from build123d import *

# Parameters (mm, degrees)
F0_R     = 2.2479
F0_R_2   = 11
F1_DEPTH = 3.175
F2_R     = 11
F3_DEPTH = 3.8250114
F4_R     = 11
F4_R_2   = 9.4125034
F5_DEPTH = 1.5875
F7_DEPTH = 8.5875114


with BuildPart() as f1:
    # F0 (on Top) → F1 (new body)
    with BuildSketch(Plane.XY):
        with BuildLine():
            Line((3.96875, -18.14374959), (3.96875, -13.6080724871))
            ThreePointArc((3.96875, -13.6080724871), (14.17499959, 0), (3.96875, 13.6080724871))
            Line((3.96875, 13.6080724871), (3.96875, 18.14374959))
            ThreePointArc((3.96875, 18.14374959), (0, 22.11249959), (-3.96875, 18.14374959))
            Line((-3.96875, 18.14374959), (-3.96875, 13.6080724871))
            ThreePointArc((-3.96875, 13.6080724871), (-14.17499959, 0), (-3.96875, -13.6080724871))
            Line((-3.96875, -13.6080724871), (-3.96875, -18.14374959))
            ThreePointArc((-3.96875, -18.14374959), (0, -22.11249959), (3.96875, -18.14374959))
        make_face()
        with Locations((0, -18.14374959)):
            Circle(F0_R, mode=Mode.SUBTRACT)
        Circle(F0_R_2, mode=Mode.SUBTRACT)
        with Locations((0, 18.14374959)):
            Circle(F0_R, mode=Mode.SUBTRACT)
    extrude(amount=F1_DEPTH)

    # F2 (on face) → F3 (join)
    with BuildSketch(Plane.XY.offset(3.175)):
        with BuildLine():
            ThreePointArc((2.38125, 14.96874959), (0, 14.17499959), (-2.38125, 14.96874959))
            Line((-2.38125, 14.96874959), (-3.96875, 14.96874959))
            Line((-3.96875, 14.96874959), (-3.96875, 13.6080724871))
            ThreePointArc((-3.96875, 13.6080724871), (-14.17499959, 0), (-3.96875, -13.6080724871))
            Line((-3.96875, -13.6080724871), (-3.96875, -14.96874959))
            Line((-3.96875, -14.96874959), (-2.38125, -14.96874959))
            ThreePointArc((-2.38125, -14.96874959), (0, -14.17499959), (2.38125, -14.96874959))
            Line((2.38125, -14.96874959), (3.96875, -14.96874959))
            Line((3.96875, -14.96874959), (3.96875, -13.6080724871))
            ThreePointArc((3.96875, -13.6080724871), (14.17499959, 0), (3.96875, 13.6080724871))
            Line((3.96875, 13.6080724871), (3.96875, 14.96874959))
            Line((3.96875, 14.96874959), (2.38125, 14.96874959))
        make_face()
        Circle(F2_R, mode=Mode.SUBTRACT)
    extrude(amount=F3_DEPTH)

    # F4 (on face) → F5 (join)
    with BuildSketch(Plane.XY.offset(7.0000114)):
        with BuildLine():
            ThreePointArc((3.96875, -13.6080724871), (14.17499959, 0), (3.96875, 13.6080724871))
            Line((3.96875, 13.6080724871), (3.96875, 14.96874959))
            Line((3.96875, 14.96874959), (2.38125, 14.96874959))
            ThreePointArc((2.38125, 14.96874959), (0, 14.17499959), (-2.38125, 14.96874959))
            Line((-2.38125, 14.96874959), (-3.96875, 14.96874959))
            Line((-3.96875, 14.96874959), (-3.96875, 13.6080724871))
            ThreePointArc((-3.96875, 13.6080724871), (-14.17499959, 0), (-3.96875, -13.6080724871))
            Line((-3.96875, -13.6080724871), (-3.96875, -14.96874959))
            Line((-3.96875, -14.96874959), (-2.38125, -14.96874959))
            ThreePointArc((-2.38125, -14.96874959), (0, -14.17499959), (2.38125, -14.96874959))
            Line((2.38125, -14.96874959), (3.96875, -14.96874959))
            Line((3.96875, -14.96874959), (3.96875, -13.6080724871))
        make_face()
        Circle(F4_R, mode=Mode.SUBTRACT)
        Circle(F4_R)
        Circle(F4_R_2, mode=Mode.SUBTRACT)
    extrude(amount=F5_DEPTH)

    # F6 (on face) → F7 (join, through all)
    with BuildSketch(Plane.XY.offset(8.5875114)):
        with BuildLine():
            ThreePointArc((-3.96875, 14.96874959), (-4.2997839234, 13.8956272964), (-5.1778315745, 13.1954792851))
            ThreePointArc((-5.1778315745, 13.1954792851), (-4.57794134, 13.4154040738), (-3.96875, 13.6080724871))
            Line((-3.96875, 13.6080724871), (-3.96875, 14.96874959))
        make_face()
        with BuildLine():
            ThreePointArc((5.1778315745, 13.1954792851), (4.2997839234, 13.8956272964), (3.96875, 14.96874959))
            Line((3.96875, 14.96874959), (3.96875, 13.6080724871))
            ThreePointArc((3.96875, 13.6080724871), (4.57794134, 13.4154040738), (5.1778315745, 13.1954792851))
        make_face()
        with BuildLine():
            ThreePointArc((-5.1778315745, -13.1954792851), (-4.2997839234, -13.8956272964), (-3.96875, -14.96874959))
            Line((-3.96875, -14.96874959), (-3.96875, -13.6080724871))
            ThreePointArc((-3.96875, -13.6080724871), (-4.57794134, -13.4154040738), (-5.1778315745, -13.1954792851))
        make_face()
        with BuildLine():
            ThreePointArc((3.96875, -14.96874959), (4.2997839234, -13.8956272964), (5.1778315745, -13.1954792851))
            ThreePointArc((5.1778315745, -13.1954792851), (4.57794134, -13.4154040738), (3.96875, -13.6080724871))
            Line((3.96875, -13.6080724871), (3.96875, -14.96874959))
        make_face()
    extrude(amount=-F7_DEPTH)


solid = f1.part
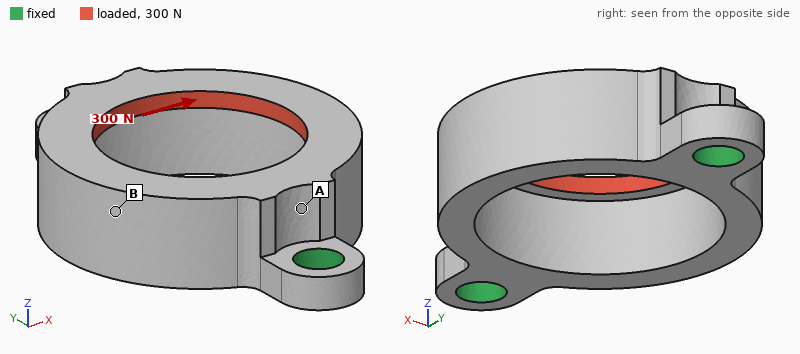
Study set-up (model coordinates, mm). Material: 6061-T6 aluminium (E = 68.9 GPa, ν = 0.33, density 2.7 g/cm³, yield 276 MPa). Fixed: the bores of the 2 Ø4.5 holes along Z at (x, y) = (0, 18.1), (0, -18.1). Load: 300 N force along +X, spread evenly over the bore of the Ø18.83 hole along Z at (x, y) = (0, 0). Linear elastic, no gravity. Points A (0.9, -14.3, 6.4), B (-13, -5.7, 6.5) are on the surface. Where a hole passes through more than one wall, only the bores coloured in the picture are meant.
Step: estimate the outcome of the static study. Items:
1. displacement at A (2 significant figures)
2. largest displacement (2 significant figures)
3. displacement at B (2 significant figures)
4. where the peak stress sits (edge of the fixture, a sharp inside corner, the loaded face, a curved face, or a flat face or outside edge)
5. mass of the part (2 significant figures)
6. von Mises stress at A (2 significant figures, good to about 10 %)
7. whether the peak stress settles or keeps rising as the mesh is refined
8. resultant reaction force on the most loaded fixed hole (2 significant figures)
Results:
7.3 µm
23 µm
20 µm
edge of the fixture
7.2 g
16 MPa
keeps rising
150 N
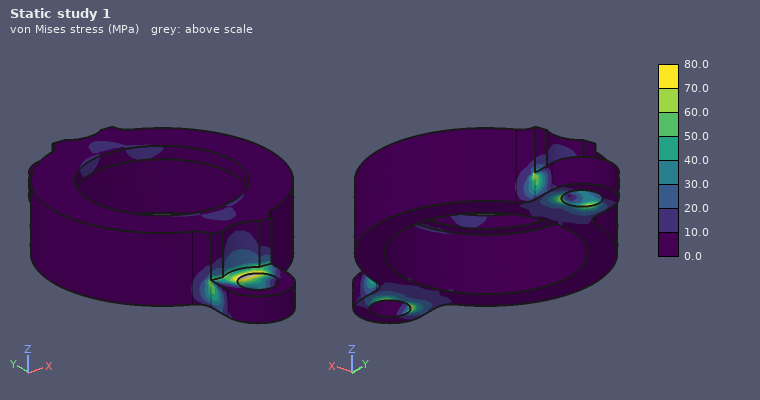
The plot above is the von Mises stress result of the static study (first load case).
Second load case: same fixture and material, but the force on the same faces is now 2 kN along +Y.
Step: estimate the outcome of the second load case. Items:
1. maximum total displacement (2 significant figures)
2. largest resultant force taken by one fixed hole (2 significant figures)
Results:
21 µm
1.1 kN
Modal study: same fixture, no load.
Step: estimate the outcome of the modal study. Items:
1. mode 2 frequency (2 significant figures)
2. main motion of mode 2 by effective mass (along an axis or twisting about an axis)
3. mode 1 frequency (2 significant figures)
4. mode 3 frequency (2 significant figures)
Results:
13 kHz
along Z
7600 Hz
20 kHz
